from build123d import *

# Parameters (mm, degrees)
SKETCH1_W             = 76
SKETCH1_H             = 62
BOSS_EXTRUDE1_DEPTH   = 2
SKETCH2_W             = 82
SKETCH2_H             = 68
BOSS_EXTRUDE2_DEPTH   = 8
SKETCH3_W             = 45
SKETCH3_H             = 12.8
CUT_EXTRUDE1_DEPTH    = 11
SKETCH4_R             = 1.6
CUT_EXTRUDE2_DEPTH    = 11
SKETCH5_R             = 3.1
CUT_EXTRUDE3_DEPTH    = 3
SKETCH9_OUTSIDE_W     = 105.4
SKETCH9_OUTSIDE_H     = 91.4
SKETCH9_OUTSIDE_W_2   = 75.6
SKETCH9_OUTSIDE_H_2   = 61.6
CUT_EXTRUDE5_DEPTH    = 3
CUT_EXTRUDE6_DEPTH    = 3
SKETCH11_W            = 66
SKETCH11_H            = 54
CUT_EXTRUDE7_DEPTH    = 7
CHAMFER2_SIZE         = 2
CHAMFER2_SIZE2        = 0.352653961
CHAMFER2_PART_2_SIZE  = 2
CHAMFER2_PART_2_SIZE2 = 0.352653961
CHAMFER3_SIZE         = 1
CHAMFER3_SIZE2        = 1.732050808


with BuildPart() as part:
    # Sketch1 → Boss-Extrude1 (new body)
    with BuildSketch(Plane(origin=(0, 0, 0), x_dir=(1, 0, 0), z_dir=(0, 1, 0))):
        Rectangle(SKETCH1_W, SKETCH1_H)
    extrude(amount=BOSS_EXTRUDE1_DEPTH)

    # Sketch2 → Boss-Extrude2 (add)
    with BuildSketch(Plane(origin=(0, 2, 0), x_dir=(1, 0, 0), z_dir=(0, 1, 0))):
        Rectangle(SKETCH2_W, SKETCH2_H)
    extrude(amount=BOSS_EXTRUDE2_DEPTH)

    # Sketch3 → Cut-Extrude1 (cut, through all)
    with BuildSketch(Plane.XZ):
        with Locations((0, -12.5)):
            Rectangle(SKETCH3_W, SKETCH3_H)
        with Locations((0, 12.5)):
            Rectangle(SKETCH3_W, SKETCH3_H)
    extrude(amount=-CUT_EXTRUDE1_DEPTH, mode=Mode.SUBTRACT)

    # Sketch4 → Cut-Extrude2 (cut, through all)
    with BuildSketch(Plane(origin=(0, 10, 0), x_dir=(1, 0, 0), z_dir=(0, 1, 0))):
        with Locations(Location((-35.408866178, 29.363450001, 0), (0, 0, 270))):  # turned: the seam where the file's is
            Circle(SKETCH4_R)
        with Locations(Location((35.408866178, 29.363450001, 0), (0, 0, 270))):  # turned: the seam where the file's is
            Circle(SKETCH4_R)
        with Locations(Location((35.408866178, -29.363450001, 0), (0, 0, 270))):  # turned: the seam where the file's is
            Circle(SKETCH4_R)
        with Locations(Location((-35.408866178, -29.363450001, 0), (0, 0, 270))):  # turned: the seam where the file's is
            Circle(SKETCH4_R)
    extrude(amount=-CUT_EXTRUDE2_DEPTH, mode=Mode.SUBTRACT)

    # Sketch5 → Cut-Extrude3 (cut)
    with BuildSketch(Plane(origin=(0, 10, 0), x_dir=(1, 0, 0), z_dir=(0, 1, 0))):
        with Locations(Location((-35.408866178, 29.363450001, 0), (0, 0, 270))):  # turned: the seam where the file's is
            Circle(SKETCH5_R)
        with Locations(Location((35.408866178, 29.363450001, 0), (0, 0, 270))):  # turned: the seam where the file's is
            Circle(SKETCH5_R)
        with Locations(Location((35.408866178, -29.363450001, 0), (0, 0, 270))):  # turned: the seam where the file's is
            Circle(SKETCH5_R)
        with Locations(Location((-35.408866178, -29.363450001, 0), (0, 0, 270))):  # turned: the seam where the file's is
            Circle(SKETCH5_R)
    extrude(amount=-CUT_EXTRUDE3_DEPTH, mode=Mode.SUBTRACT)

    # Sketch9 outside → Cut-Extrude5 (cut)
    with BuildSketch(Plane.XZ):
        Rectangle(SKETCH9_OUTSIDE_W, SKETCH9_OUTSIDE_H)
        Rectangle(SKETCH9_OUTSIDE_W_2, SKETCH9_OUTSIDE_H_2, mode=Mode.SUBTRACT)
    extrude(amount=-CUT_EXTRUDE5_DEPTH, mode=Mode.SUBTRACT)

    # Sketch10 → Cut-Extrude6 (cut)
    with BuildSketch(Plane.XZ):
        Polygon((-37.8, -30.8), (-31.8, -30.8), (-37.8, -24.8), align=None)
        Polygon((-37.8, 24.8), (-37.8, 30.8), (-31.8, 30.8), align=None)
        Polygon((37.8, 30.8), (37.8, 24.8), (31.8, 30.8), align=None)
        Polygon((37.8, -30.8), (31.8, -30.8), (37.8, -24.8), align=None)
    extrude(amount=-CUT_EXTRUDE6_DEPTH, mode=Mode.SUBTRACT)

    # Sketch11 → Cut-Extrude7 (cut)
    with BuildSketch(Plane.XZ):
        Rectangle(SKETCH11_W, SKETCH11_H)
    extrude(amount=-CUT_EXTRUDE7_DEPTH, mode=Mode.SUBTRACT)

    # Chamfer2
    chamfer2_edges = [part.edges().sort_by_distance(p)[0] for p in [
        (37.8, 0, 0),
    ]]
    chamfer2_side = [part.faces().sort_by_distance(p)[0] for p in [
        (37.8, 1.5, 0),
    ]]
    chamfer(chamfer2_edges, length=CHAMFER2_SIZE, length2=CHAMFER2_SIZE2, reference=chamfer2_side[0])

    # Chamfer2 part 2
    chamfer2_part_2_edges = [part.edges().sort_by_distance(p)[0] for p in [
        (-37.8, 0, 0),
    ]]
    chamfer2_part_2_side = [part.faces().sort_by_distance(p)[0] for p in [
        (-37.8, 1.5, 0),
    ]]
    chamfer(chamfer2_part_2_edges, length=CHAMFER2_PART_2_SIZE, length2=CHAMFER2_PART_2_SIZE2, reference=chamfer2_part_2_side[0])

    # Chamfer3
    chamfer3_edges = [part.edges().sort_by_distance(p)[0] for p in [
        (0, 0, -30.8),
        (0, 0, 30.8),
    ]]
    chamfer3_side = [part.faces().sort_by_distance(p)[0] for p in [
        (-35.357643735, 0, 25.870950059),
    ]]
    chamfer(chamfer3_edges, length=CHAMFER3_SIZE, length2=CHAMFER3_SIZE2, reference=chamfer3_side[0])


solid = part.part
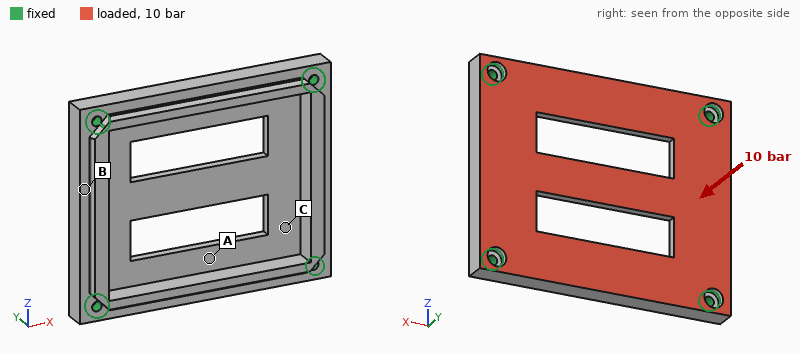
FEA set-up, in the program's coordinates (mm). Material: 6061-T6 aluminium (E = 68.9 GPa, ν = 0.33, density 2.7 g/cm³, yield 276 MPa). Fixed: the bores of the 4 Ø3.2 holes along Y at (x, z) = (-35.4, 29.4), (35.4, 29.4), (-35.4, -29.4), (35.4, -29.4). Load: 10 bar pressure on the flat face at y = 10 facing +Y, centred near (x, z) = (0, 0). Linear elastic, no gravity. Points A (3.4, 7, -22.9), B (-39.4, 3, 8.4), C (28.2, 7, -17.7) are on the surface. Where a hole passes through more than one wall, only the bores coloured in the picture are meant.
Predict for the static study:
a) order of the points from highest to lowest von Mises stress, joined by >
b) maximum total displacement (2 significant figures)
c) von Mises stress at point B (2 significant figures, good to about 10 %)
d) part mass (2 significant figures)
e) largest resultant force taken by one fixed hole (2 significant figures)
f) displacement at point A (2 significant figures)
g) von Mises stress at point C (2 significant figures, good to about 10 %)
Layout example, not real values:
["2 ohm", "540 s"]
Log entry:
["C > B > A", "0.36 mm", "26 MPa", "64 g", "1.3 kN", "0.082 mm", "49 MPa"]
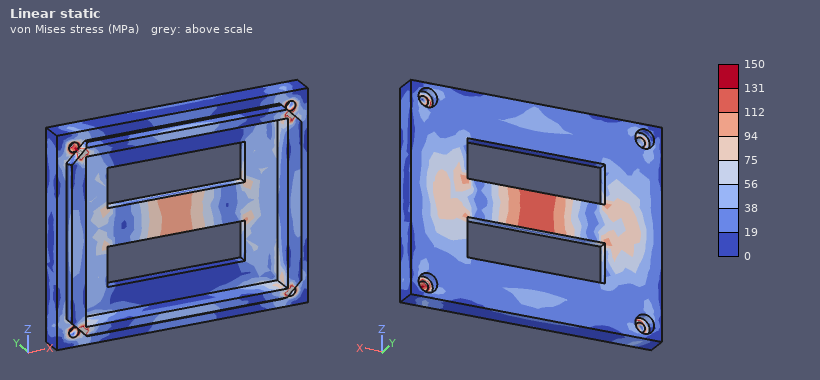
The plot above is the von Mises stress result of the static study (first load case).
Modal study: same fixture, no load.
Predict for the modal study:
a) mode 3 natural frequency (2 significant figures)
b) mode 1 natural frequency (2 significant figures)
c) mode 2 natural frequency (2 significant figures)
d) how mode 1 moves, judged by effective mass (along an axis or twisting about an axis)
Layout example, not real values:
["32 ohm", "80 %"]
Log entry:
["6800 Hz", "3700 Hz", "6800 Hz", "along Y"]
